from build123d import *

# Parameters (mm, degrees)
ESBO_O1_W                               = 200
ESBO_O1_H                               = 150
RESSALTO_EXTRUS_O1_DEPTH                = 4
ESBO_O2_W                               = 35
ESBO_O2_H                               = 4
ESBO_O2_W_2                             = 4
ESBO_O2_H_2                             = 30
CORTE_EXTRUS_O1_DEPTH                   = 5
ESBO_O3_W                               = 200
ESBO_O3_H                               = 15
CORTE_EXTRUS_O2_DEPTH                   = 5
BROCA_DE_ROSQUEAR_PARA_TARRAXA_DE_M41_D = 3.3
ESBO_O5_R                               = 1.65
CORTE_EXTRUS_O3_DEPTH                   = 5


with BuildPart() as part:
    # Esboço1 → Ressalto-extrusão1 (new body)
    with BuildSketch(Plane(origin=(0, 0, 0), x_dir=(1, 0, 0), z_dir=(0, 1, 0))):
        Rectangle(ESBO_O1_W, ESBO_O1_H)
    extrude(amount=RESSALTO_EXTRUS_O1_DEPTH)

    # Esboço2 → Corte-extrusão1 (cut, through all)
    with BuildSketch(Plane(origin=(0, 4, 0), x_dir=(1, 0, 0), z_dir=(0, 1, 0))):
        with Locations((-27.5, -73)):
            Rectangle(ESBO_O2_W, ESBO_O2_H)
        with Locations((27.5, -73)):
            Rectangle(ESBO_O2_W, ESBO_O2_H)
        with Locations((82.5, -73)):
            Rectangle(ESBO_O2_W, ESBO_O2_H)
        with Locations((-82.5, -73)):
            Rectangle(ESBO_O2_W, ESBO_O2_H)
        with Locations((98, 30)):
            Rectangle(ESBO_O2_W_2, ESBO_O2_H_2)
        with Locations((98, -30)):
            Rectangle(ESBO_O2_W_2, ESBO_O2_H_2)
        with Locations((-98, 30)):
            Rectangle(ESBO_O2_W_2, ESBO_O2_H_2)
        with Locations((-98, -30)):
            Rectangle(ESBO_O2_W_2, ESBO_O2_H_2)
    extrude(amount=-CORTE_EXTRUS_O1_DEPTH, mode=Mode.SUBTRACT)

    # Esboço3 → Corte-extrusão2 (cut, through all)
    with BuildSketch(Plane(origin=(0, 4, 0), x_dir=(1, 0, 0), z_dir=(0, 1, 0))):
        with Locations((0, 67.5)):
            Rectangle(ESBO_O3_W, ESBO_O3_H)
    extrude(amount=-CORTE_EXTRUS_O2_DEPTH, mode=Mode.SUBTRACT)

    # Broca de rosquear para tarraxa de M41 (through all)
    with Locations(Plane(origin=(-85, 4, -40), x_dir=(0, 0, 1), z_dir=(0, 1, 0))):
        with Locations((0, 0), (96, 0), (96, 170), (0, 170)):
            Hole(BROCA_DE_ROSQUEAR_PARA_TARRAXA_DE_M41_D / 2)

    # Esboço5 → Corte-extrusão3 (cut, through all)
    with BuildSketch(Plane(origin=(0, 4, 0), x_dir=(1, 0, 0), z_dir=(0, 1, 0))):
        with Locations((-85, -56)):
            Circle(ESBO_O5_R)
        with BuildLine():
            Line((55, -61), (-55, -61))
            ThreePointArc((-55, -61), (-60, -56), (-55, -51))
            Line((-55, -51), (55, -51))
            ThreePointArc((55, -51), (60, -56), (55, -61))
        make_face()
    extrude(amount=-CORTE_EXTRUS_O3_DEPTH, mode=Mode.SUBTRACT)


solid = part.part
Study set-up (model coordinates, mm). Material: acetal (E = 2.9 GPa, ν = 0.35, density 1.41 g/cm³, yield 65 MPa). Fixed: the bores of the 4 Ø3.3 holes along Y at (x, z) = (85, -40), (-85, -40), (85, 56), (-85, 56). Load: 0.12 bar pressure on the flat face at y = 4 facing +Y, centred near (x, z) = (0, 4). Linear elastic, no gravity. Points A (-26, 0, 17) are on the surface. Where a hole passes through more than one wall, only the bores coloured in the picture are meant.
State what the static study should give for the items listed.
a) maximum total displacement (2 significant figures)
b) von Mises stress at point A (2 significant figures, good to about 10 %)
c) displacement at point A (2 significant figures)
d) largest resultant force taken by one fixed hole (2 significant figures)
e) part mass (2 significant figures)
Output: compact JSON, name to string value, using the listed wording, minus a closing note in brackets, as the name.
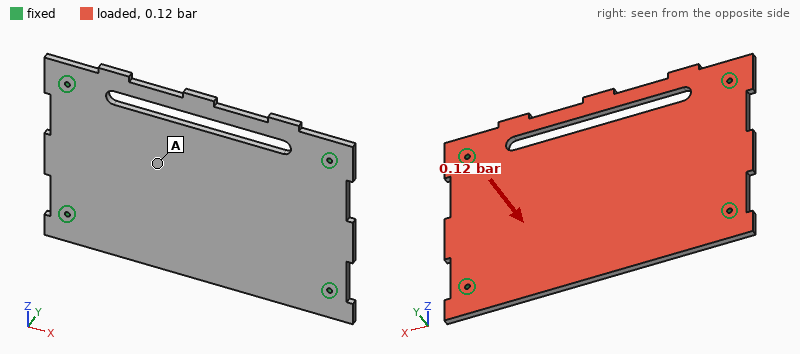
{"maximum total displacement": "2.6 mm", "von Mises stress at point A": "4.6 MPa", "displacement at point A": "2.2 mm", "largest resultant force taken by one fixed hole": "79 N", "part mass": "140 g"}
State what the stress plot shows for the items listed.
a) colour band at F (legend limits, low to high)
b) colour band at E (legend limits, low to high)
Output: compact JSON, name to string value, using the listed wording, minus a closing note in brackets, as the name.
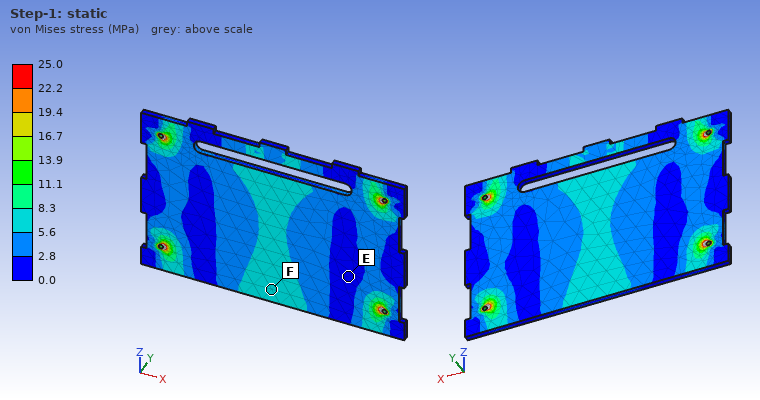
{"colour band at F": "5.6 to 8.3 MPa", "colour band at E": "0.0 to 2.8 MPa"}
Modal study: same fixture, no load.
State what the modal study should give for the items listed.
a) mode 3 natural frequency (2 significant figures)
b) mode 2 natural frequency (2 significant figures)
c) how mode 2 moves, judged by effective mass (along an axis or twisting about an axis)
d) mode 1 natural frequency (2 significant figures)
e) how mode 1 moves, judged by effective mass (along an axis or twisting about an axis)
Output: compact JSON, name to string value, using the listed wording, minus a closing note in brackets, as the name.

{"mode 3 natural frequency": "300 Hz", "mode 2 natural frequency": "250 Hz", "how mode 2 moves, judged by effective mass": "twisting about X", "mode 1 natural frequency": "170 Hz", "how mode 1 moves, judged by effective mass": "along Y"}
